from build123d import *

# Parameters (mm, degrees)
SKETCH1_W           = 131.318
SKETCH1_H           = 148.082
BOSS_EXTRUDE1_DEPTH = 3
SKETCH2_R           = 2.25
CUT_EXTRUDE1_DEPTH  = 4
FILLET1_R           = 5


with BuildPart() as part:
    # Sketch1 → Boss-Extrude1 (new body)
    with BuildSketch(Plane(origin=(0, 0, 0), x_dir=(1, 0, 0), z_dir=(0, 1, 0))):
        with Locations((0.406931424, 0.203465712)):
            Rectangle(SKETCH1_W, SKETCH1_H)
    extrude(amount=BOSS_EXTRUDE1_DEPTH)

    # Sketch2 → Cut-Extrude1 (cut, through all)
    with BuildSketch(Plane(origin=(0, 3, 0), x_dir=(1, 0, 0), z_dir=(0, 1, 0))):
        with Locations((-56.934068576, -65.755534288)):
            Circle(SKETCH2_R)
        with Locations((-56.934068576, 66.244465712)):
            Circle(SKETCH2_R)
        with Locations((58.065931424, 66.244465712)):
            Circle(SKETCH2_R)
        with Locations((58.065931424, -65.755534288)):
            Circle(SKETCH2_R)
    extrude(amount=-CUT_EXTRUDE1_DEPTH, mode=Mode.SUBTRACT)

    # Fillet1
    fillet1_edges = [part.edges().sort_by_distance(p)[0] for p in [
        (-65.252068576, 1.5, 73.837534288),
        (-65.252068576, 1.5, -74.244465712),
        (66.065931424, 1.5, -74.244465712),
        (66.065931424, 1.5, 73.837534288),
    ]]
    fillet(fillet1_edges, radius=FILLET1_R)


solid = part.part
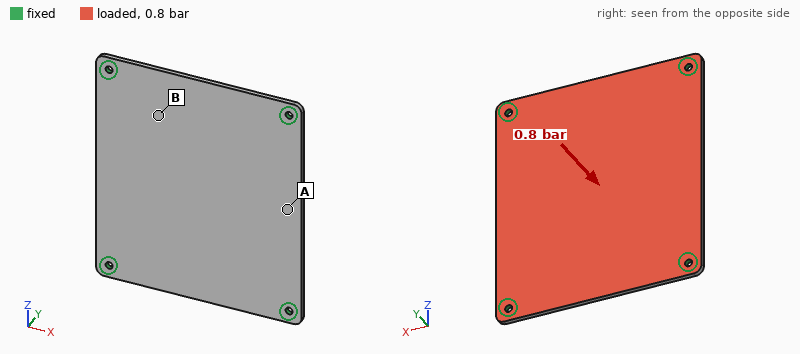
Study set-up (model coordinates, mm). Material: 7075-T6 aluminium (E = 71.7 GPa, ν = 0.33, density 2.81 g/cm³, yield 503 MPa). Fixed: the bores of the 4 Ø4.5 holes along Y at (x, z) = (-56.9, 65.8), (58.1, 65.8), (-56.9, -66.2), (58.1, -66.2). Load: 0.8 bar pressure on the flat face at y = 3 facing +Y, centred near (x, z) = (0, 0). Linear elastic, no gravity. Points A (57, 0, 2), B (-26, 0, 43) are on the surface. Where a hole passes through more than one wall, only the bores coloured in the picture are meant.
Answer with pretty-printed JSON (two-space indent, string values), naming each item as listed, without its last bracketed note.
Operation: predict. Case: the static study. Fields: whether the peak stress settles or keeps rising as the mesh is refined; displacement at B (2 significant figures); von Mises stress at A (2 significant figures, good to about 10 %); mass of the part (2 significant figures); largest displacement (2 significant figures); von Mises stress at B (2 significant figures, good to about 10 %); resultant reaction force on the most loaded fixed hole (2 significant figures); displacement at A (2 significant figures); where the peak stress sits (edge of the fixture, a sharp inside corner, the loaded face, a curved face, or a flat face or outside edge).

{
  "whether the peak stress settles or keeps rising as the mesh is refined": "keeps rising",
  "displacement at B": "0.49 mm",
  "von Mises stress at A": "54 MPa",
  "mass of the part": "160 g",
  "largest displacement": "0.89 mm",
  "von Mises stress at B": "26 MPa",
  "resultant reaction force on the most loaded fixed hole": "390 N",
  "displacement at A": "0.62 mm",
  "where the peak stress sits": "edge of the fixture"
}
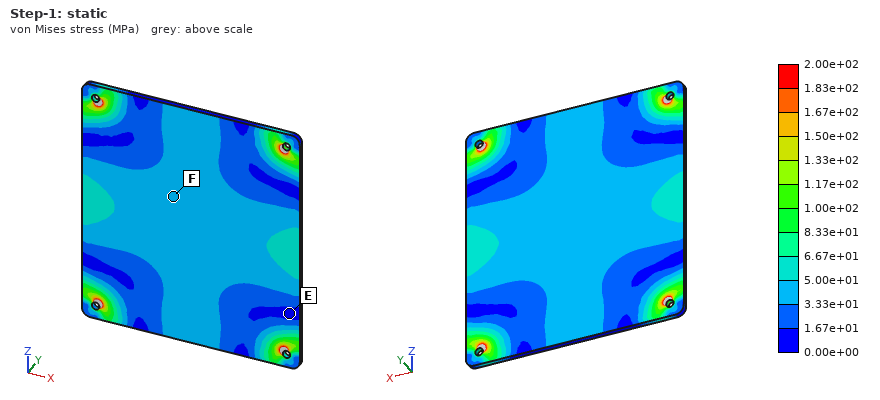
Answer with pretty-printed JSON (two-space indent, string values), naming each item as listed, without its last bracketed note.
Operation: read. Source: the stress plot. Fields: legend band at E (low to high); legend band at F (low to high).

{
  "legend band at E": "0.00e+00 to 1.67e+01 MPa",
  "legend band at F": "3.33e+01 to 5.00e+01 MPa"
}
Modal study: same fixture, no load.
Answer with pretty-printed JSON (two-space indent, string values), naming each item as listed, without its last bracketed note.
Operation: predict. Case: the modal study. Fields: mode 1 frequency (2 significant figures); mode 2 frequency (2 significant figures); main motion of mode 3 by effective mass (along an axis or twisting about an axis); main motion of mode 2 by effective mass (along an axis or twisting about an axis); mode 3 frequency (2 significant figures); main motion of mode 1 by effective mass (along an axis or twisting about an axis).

{
  "mode 1 frequency": "630 Hz",
  "mode 2 frequency": "1000 Hz",
  "main motion of mode 3 by effective mass": "twisting about X",
  "main motion of mode 2 by effective mass": "twisting about Z",
  "mode 3 frequency": "1200 Hz",
  "main motion of mode 1 by effective mass": "along Y"
}
